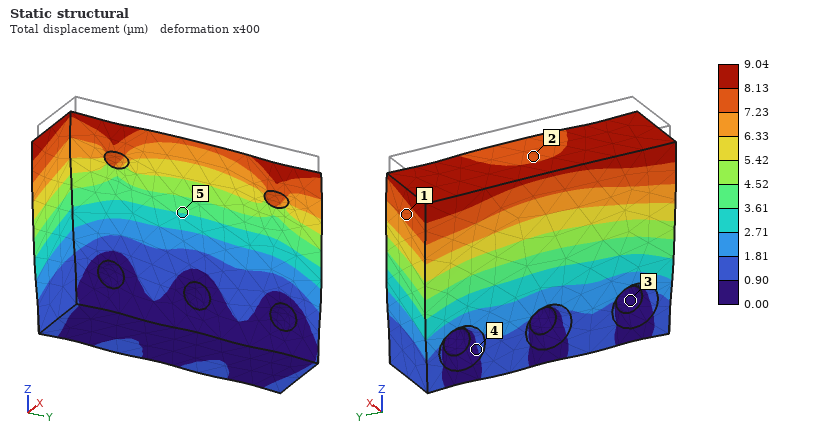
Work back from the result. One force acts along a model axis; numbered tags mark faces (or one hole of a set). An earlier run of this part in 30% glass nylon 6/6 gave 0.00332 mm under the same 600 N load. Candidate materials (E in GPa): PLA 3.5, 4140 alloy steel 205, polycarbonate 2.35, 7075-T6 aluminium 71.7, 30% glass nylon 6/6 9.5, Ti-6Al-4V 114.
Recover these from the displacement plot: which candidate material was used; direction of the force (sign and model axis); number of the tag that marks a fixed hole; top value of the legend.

PLA
-Z
3
9.04 µm
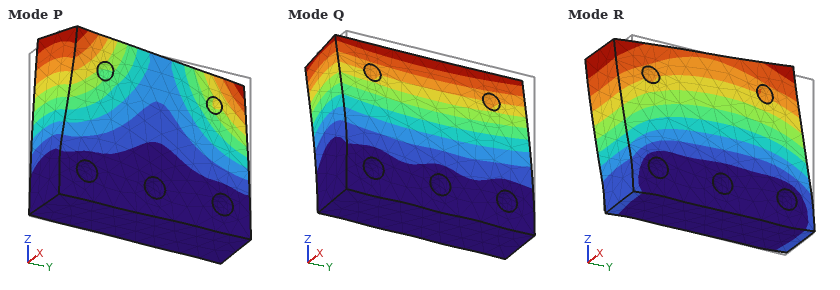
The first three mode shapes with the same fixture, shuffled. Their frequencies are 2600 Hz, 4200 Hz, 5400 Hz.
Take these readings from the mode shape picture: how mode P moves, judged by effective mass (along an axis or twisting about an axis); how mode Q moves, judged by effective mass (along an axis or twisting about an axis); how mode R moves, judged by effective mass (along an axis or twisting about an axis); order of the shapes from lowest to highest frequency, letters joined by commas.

twisting about Z
along X
along Y
Q, P, R
